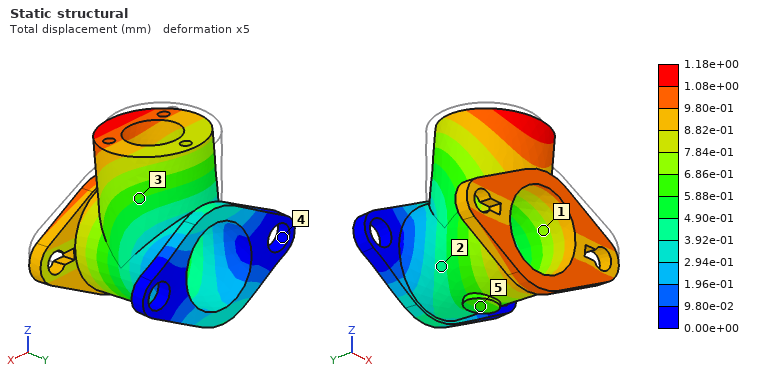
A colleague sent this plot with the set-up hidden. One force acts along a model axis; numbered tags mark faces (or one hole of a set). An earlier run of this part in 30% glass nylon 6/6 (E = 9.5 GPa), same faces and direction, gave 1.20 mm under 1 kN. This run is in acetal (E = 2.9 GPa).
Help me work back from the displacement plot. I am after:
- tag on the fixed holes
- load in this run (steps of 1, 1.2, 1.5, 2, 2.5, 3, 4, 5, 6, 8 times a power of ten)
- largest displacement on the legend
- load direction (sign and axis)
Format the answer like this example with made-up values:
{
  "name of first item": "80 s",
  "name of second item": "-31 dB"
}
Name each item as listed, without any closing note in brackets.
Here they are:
{
  "tag on the fixed holes": "4",
  "load in this run": "300 N",
  "largest displacement on the legend": "1.18e+00 mm",
  "load direction": "-Z"
}
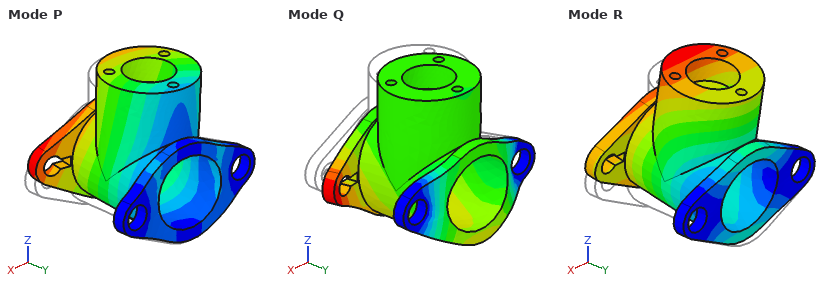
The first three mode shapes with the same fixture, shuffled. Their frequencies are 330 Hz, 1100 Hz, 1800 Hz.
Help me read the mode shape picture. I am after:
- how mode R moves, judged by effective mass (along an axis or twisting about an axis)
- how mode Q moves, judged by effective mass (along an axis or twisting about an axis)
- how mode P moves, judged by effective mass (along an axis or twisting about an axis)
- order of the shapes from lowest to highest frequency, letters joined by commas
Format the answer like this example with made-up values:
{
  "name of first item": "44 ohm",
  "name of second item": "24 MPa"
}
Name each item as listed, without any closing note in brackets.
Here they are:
{
  "how mode R moves, judged by effective mass": "along Z",
  "how mode Q moves, judged by effective mass": "along Y",
  "how mode P moves, judged by effective mass": "along X",
  "order of the shapes from lowest to highest frequency, letters joined by commas": "R, P, Q"
}
